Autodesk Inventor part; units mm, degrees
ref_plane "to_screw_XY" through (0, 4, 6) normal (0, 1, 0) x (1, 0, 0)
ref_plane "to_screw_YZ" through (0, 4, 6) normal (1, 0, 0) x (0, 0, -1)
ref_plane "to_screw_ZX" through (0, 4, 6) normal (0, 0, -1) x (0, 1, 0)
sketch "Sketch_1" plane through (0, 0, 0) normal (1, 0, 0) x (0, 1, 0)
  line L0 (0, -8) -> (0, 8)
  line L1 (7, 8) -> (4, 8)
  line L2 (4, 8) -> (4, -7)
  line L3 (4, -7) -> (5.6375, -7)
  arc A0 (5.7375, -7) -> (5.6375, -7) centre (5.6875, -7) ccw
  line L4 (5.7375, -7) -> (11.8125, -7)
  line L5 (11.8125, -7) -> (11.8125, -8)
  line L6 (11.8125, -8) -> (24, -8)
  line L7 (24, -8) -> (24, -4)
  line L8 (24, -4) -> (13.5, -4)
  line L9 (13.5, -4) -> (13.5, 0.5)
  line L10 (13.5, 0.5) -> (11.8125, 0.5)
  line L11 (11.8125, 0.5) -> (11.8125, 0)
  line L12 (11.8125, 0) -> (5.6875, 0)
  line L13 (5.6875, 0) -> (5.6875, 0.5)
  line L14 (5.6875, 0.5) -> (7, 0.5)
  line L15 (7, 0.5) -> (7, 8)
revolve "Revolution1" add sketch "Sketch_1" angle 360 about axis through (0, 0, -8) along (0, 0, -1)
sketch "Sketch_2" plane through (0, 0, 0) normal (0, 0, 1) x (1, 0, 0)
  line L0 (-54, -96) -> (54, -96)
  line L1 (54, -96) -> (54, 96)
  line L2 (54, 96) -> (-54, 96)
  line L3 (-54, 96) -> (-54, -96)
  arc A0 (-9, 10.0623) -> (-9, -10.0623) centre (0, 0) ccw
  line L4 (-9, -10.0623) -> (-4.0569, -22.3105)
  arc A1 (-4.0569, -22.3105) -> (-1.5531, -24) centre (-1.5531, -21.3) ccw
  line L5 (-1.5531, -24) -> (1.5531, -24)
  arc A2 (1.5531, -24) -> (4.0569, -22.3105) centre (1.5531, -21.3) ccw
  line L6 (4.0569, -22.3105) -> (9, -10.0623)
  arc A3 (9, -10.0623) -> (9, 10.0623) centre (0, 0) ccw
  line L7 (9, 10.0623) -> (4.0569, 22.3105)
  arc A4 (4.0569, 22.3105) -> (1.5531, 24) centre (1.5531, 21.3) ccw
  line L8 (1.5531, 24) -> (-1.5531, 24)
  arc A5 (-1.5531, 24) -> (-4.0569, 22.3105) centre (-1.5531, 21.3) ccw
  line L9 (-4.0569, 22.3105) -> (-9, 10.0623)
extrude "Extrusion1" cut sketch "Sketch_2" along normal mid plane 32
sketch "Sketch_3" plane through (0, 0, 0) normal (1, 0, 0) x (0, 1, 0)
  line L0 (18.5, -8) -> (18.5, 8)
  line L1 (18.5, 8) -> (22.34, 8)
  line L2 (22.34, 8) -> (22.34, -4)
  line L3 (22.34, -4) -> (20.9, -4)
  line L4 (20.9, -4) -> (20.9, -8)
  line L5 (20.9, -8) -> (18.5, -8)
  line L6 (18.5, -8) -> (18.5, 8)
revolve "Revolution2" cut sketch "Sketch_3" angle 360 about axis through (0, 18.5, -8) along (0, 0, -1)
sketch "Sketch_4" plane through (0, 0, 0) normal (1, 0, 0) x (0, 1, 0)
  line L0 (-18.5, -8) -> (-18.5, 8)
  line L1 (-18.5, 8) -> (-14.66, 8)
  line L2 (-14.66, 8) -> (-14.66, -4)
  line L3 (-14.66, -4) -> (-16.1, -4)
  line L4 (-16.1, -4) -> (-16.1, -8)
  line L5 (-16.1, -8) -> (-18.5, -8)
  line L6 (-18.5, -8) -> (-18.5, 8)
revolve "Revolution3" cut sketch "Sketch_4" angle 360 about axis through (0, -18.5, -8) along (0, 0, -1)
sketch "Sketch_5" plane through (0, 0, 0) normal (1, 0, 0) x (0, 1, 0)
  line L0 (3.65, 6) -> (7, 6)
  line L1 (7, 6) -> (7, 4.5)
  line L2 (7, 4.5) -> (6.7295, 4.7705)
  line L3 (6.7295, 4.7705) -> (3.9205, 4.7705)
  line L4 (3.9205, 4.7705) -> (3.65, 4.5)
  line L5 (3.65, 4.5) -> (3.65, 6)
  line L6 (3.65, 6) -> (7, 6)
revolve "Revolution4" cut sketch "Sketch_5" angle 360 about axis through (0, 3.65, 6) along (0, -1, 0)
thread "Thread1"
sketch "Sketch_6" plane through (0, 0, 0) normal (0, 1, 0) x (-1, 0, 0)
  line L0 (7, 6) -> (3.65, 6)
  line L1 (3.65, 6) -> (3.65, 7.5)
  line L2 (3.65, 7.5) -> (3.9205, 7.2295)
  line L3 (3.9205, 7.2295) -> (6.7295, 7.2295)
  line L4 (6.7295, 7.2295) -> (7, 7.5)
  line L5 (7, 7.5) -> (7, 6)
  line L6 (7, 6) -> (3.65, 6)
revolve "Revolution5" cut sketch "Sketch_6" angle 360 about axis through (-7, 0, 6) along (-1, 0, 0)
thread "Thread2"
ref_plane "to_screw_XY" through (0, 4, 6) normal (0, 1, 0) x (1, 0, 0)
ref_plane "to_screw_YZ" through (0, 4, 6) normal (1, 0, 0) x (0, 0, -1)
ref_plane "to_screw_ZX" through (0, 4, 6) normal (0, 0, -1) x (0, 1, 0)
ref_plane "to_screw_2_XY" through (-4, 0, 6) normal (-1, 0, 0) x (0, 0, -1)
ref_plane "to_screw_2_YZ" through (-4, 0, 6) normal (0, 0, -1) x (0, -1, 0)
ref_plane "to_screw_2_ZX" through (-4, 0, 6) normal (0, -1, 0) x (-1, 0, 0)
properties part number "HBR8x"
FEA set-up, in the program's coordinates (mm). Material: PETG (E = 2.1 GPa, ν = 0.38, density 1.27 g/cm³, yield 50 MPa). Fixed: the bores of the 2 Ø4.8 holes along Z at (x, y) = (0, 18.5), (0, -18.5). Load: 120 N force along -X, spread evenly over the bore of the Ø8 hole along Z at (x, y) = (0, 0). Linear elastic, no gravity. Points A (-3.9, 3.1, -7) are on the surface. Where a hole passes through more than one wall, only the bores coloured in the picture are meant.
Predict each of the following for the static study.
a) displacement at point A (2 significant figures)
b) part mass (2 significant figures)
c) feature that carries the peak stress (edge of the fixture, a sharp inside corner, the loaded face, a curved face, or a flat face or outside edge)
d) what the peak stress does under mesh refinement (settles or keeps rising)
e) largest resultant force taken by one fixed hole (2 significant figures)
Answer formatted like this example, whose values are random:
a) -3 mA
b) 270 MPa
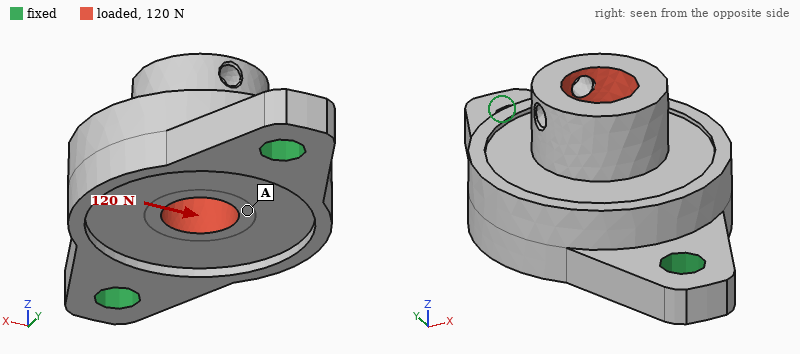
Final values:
a) 0.039 mm
b) 7.0 g
c) edge of the fixture
d) keeps rising
e) 60 N
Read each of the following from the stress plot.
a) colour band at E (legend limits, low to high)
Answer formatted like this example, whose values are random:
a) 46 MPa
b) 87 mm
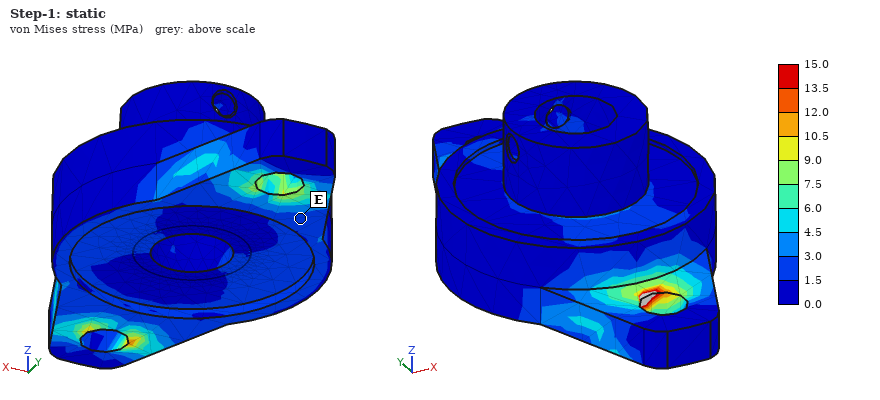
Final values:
a) 1.5 to 3.0 MPa
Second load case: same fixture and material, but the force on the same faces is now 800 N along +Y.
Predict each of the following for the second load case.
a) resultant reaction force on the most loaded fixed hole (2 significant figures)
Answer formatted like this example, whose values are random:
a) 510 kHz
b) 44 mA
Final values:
a) 430 N
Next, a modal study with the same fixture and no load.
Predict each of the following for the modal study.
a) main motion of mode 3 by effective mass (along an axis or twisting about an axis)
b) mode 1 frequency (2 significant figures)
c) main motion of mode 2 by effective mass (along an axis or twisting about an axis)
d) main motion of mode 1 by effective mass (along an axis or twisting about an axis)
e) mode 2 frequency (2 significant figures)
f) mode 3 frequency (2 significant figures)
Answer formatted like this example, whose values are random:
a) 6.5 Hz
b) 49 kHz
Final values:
a) along X
b) 2100 Hz
c) along Z
d) along X
e) 3700 Hz
f) 6500 Hz
